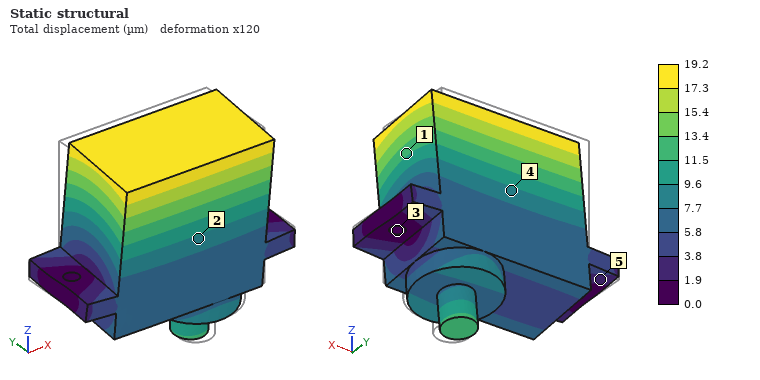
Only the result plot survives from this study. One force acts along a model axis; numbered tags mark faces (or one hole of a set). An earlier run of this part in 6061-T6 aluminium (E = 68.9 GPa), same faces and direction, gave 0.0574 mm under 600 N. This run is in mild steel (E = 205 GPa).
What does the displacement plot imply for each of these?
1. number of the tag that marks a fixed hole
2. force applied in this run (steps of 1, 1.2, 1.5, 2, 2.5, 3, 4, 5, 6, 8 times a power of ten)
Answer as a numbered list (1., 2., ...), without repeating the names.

1. 3
2. 600 N
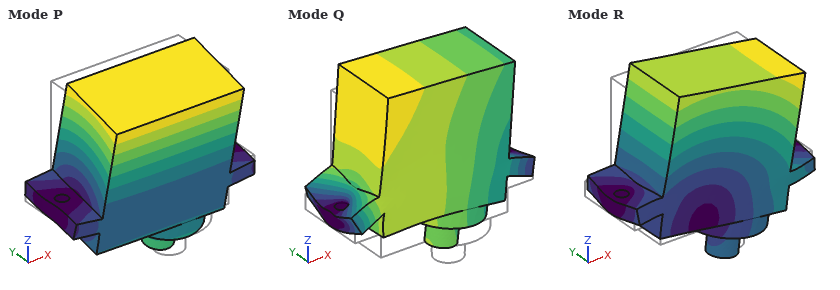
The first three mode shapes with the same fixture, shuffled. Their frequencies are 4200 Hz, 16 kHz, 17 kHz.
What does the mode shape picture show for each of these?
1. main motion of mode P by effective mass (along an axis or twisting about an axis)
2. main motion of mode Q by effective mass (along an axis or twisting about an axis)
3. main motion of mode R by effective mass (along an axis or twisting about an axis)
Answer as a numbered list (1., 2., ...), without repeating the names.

1. along Y
2. along Z
3. along X
